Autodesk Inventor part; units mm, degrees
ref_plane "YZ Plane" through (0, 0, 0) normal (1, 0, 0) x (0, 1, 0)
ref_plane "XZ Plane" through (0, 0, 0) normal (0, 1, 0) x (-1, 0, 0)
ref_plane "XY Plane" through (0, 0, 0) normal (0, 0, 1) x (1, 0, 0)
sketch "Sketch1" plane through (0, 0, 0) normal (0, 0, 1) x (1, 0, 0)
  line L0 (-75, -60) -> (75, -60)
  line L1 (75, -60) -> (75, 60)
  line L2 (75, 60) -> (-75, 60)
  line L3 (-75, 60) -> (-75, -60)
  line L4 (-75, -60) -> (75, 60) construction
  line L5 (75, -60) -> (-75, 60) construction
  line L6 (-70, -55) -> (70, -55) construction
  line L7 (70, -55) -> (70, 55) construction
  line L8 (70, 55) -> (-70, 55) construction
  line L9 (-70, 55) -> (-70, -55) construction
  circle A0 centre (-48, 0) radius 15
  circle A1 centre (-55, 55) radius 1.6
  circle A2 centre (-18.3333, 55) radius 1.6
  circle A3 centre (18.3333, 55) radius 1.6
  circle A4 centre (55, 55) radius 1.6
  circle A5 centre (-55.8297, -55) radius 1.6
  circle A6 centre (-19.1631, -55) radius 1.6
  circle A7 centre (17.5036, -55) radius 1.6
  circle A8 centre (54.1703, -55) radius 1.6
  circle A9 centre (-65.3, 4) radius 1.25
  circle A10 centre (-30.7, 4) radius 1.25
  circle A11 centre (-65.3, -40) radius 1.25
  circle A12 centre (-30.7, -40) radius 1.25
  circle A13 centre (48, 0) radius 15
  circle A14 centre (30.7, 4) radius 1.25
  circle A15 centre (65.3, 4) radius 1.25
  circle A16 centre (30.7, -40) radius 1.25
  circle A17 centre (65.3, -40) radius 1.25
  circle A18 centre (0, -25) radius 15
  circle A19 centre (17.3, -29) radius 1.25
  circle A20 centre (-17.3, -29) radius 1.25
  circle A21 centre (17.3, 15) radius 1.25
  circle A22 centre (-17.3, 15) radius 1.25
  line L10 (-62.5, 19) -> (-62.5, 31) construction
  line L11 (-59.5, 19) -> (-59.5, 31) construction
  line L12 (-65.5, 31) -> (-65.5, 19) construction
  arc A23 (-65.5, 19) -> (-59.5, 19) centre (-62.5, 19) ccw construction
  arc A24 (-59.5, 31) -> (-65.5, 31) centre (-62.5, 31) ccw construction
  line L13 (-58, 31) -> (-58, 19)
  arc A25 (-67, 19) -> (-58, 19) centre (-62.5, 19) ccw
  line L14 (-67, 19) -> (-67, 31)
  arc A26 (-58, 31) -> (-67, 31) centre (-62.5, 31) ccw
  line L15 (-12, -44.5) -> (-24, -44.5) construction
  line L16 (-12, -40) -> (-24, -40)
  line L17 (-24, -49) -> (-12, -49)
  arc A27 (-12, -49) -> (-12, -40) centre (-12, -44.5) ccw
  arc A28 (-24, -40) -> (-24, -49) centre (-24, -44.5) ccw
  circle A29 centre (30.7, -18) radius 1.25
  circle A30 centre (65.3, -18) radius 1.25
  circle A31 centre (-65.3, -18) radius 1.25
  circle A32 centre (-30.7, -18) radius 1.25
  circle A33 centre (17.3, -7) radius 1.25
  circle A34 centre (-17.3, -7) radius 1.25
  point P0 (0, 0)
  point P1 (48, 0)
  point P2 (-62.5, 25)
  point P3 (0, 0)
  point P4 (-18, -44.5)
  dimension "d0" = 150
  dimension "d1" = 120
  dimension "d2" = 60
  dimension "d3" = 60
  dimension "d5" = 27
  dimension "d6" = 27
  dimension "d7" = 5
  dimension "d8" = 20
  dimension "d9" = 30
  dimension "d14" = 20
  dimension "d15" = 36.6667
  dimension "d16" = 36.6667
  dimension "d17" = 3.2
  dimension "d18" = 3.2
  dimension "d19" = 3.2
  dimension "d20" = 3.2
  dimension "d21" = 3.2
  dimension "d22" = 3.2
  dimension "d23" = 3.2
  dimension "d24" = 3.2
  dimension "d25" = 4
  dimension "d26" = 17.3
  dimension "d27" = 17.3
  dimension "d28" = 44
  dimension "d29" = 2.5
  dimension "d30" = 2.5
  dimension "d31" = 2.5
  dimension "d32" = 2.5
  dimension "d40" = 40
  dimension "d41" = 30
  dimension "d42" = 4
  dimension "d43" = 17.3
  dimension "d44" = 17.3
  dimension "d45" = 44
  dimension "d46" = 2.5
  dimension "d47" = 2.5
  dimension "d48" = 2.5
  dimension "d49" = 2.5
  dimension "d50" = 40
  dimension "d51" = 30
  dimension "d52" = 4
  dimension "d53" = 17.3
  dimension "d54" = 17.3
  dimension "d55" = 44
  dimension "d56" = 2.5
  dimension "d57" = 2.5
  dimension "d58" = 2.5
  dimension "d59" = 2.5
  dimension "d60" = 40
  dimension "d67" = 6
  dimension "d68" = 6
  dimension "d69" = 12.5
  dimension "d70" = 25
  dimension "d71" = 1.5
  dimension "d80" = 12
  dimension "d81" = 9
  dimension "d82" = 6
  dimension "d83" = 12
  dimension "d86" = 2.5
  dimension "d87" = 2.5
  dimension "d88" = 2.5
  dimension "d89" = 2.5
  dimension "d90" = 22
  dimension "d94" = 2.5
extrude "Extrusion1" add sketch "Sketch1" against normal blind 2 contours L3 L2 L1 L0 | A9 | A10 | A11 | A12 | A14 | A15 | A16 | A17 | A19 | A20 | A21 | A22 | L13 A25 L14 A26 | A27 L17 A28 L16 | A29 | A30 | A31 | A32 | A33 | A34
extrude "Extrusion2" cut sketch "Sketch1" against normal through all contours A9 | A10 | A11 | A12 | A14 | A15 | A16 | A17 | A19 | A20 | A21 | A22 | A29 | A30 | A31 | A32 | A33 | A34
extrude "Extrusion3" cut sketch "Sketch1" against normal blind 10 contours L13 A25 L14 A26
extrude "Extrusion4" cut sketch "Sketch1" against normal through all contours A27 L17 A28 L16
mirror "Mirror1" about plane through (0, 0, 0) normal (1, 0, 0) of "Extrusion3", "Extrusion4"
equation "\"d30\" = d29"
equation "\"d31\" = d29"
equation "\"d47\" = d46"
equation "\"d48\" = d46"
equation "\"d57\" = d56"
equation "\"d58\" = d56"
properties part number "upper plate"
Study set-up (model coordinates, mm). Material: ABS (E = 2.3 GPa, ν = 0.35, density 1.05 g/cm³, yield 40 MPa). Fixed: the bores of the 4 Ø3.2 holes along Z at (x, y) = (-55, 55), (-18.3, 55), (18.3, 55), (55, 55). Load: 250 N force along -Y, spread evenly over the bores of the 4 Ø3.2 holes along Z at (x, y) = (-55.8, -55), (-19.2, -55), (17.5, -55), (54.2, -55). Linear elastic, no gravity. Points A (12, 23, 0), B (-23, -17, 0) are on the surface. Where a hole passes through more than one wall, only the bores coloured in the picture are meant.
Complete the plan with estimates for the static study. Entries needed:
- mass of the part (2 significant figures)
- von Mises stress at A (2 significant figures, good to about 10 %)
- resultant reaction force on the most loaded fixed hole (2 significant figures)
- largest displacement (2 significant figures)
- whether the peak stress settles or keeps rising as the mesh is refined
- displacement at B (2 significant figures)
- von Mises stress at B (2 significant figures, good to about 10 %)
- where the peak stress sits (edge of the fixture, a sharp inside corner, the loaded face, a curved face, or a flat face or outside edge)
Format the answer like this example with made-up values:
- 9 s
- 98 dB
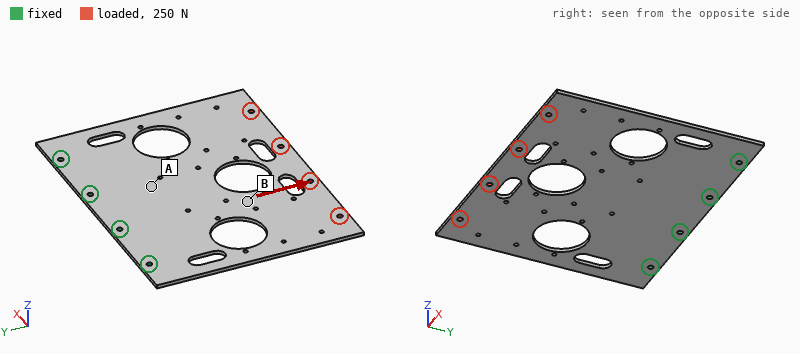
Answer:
- 32 g
- 0.99 MPa
- 65 N
- 0.16 mm
- keeps rising
- 0.056 mm
- 2.2 MPa
- a sharp inside corner
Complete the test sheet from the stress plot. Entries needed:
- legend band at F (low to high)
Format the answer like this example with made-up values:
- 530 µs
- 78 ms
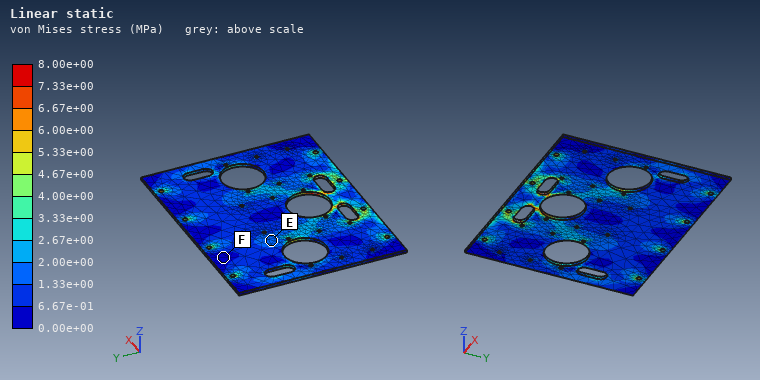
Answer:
- 0.00e+00 to 6.67e-01 MPa
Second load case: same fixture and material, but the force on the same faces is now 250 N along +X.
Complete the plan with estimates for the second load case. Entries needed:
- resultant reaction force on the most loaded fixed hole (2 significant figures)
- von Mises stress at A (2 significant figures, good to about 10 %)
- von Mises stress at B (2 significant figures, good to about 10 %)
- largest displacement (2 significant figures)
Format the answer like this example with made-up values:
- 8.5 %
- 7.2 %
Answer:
- 230 N
- 2.4 MPa
- 4.0 MPa
- 0.55 mm
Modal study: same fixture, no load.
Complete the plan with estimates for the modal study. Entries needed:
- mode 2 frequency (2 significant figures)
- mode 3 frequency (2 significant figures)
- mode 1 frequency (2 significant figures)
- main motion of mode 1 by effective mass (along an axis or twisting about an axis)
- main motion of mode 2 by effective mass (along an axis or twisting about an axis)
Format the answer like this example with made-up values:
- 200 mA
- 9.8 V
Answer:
- 65 Hz
- 160 Hz
- 35 Hz
- along Z
- twisting about Y
